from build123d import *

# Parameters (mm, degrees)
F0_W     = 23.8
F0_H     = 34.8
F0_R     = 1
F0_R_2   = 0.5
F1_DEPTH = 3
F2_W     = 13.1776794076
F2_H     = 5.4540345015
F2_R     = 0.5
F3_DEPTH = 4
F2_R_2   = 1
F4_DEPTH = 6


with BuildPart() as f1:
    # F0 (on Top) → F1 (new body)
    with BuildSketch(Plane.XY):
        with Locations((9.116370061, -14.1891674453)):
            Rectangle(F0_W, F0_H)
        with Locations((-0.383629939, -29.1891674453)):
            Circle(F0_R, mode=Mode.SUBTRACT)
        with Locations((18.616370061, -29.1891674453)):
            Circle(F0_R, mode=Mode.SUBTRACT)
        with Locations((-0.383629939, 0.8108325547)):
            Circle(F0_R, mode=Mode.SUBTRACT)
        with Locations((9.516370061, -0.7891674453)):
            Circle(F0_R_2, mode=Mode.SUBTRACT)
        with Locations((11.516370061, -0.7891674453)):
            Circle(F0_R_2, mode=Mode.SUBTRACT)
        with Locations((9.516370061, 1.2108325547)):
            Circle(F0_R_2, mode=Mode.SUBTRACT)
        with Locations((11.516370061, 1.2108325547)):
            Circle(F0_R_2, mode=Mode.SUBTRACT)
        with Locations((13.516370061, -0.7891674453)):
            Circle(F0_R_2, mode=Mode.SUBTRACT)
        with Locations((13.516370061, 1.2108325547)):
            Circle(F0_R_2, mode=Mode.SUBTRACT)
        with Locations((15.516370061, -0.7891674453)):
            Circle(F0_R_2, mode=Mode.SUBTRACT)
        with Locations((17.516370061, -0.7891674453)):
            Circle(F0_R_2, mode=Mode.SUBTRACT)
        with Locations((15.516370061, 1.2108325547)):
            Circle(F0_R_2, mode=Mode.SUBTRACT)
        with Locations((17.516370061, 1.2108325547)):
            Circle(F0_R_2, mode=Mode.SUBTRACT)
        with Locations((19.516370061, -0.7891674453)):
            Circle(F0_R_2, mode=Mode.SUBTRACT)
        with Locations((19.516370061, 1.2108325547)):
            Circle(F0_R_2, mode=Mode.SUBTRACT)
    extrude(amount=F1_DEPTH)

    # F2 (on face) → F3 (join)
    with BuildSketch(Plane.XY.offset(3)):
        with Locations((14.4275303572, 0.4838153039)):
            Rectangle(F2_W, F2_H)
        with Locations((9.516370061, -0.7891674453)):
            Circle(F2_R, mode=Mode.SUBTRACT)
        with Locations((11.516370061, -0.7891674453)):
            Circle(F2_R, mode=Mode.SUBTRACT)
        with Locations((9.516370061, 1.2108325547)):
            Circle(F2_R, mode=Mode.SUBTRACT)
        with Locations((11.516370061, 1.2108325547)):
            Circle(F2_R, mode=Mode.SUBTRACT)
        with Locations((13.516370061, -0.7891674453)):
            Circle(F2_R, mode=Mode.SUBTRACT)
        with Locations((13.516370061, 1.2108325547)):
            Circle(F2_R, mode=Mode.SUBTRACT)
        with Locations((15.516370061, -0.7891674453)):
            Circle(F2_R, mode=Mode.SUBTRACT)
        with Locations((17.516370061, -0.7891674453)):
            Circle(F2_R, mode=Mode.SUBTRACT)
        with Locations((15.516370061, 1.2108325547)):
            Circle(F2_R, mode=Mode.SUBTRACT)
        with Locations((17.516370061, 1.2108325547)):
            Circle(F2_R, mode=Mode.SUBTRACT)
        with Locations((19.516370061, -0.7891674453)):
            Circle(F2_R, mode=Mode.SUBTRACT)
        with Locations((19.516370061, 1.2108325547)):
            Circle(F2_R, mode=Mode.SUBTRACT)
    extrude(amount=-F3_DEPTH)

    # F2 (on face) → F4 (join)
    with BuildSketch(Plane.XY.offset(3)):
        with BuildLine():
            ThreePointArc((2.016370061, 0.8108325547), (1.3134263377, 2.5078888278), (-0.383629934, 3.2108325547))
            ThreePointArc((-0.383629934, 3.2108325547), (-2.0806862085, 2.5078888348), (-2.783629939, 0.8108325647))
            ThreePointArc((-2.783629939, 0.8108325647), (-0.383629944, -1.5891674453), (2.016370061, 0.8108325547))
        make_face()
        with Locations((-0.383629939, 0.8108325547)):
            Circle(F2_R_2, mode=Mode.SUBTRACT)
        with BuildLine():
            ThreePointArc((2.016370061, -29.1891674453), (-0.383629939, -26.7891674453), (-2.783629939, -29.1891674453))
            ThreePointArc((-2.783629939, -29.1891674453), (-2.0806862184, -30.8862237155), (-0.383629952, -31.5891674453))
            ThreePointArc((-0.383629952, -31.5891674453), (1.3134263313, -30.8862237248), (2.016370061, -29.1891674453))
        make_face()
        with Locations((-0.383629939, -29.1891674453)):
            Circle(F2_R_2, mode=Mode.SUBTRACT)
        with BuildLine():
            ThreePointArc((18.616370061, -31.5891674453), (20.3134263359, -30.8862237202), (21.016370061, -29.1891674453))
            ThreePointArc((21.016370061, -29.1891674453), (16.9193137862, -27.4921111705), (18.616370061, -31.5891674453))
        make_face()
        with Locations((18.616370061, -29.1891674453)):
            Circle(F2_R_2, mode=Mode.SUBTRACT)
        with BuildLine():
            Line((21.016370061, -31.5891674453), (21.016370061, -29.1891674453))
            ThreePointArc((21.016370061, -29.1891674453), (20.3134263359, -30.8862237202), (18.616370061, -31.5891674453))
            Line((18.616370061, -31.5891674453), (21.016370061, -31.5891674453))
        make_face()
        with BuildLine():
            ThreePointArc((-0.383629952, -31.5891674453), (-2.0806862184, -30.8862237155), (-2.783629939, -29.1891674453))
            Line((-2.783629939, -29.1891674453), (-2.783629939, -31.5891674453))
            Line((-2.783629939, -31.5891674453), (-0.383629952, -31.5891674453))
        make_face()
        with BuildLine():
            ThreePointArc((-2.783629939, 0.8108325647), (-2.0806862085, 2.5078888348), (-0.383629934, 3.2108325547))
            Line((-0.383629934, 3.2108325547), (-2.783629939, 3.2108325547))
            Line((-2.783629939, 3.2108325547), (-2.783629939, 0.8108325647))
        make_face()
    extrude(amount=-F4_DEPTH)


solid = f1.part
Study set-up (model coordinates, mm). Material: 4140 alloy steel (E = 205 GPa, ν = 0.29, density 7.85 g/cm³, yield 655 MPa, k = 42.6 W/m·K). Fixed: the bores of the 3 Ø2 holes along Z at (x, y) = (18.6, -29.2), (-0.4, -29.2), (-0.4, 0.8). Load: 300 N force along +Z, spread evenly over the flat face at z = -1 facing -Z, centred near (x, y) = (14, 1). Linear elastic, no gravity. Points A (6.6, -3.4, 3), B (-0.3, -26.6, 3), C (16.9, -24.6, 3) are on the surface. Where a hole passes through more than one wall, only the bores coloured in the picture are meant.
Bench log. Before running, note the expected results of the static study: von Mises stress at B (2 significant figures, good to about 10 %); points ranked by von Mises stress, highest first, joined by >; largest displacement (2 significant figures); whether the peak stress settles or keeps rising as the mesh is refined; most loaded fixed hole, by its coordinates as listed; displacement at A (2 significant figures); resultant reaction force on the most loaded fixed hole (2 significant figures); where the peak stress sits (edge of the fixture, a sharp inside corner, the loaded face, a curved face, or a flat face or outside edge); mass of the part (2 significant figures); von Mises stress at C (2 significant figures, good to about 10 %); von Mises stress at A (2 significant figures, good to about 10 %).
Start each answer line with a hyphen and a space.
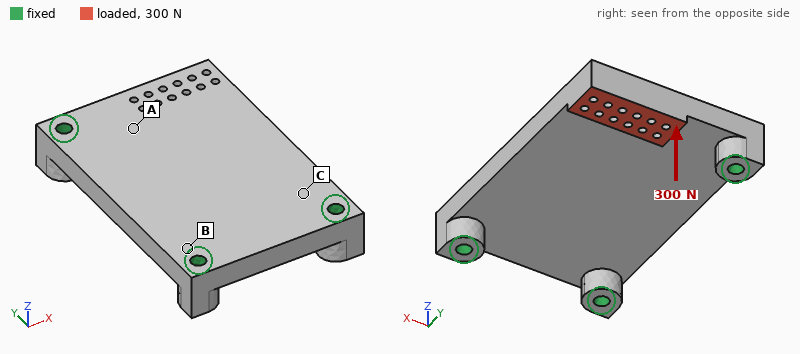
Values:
- 17 MPa
- A > C > B
- 59 µm
- keeps rising
- (-0.4, 0.8)
- 10 µm
- 270 N
- edge of the fixture
- 21 g
- 47 MPa
- 68 MPa
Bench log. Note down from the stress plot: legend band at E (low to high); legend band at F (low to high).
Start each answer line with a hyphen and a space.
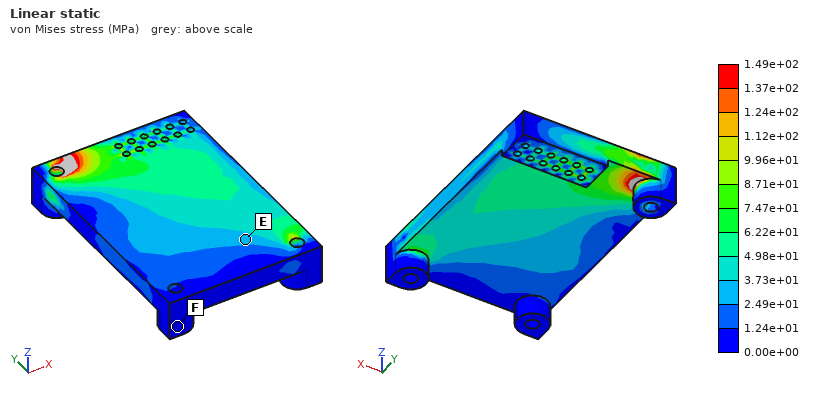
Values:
- 2.49e+01 to 3.73e+01 MPa
- 0.00e+00 to 1.24e+01 MPa
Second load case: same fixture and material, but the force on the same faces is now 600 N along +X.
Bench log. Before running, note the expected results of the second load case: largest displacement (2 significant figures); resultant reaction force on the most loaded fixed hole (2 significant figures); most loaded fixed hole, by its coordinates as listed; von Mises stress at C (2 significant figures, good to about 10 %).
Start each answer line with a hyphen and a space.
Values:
- 28 µm
- 540 N
- (-0.4, 0.8)
- 25 MPa
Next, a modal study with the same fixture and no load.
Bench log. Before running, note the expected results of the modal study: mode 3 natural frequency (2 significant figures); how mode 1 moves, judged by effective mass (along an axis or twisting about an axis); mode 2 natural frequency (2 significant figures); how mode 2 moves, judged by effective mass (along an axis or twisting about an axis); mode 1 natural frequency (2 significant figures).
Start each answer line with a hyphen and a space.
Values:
- 22 kHz
- along Z
- 15 kHz
- along Z
- 6900 Hz
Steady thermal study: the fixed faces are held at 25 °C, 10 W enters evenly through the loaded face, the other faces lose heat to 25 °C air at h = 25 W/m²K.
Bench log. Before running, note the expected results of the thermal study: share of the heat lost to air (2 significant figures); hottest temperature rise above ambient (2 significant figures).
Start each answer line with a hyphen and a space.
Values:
- 12 %
- 77 K
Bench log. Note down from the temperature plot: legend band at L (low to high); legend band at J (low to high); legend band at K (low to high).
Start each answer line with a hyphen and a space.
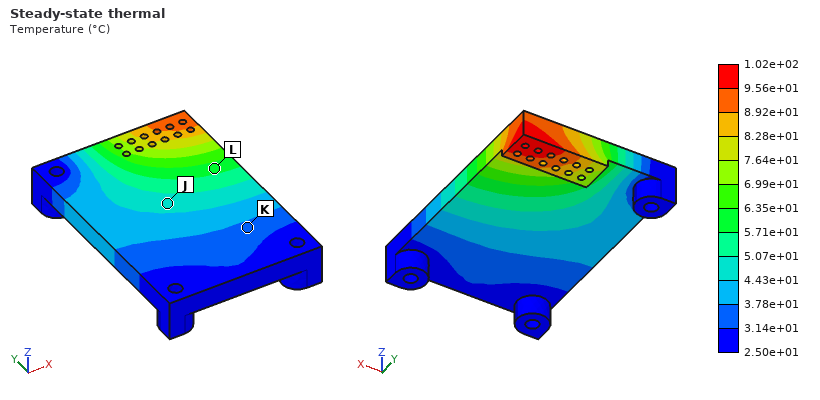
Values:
- 5.71e+01 to 6.35e+01 °C
- 4.43e+01 to 5.07e+01 °C
- 3.14e+01 to 3.78e+01 °C
